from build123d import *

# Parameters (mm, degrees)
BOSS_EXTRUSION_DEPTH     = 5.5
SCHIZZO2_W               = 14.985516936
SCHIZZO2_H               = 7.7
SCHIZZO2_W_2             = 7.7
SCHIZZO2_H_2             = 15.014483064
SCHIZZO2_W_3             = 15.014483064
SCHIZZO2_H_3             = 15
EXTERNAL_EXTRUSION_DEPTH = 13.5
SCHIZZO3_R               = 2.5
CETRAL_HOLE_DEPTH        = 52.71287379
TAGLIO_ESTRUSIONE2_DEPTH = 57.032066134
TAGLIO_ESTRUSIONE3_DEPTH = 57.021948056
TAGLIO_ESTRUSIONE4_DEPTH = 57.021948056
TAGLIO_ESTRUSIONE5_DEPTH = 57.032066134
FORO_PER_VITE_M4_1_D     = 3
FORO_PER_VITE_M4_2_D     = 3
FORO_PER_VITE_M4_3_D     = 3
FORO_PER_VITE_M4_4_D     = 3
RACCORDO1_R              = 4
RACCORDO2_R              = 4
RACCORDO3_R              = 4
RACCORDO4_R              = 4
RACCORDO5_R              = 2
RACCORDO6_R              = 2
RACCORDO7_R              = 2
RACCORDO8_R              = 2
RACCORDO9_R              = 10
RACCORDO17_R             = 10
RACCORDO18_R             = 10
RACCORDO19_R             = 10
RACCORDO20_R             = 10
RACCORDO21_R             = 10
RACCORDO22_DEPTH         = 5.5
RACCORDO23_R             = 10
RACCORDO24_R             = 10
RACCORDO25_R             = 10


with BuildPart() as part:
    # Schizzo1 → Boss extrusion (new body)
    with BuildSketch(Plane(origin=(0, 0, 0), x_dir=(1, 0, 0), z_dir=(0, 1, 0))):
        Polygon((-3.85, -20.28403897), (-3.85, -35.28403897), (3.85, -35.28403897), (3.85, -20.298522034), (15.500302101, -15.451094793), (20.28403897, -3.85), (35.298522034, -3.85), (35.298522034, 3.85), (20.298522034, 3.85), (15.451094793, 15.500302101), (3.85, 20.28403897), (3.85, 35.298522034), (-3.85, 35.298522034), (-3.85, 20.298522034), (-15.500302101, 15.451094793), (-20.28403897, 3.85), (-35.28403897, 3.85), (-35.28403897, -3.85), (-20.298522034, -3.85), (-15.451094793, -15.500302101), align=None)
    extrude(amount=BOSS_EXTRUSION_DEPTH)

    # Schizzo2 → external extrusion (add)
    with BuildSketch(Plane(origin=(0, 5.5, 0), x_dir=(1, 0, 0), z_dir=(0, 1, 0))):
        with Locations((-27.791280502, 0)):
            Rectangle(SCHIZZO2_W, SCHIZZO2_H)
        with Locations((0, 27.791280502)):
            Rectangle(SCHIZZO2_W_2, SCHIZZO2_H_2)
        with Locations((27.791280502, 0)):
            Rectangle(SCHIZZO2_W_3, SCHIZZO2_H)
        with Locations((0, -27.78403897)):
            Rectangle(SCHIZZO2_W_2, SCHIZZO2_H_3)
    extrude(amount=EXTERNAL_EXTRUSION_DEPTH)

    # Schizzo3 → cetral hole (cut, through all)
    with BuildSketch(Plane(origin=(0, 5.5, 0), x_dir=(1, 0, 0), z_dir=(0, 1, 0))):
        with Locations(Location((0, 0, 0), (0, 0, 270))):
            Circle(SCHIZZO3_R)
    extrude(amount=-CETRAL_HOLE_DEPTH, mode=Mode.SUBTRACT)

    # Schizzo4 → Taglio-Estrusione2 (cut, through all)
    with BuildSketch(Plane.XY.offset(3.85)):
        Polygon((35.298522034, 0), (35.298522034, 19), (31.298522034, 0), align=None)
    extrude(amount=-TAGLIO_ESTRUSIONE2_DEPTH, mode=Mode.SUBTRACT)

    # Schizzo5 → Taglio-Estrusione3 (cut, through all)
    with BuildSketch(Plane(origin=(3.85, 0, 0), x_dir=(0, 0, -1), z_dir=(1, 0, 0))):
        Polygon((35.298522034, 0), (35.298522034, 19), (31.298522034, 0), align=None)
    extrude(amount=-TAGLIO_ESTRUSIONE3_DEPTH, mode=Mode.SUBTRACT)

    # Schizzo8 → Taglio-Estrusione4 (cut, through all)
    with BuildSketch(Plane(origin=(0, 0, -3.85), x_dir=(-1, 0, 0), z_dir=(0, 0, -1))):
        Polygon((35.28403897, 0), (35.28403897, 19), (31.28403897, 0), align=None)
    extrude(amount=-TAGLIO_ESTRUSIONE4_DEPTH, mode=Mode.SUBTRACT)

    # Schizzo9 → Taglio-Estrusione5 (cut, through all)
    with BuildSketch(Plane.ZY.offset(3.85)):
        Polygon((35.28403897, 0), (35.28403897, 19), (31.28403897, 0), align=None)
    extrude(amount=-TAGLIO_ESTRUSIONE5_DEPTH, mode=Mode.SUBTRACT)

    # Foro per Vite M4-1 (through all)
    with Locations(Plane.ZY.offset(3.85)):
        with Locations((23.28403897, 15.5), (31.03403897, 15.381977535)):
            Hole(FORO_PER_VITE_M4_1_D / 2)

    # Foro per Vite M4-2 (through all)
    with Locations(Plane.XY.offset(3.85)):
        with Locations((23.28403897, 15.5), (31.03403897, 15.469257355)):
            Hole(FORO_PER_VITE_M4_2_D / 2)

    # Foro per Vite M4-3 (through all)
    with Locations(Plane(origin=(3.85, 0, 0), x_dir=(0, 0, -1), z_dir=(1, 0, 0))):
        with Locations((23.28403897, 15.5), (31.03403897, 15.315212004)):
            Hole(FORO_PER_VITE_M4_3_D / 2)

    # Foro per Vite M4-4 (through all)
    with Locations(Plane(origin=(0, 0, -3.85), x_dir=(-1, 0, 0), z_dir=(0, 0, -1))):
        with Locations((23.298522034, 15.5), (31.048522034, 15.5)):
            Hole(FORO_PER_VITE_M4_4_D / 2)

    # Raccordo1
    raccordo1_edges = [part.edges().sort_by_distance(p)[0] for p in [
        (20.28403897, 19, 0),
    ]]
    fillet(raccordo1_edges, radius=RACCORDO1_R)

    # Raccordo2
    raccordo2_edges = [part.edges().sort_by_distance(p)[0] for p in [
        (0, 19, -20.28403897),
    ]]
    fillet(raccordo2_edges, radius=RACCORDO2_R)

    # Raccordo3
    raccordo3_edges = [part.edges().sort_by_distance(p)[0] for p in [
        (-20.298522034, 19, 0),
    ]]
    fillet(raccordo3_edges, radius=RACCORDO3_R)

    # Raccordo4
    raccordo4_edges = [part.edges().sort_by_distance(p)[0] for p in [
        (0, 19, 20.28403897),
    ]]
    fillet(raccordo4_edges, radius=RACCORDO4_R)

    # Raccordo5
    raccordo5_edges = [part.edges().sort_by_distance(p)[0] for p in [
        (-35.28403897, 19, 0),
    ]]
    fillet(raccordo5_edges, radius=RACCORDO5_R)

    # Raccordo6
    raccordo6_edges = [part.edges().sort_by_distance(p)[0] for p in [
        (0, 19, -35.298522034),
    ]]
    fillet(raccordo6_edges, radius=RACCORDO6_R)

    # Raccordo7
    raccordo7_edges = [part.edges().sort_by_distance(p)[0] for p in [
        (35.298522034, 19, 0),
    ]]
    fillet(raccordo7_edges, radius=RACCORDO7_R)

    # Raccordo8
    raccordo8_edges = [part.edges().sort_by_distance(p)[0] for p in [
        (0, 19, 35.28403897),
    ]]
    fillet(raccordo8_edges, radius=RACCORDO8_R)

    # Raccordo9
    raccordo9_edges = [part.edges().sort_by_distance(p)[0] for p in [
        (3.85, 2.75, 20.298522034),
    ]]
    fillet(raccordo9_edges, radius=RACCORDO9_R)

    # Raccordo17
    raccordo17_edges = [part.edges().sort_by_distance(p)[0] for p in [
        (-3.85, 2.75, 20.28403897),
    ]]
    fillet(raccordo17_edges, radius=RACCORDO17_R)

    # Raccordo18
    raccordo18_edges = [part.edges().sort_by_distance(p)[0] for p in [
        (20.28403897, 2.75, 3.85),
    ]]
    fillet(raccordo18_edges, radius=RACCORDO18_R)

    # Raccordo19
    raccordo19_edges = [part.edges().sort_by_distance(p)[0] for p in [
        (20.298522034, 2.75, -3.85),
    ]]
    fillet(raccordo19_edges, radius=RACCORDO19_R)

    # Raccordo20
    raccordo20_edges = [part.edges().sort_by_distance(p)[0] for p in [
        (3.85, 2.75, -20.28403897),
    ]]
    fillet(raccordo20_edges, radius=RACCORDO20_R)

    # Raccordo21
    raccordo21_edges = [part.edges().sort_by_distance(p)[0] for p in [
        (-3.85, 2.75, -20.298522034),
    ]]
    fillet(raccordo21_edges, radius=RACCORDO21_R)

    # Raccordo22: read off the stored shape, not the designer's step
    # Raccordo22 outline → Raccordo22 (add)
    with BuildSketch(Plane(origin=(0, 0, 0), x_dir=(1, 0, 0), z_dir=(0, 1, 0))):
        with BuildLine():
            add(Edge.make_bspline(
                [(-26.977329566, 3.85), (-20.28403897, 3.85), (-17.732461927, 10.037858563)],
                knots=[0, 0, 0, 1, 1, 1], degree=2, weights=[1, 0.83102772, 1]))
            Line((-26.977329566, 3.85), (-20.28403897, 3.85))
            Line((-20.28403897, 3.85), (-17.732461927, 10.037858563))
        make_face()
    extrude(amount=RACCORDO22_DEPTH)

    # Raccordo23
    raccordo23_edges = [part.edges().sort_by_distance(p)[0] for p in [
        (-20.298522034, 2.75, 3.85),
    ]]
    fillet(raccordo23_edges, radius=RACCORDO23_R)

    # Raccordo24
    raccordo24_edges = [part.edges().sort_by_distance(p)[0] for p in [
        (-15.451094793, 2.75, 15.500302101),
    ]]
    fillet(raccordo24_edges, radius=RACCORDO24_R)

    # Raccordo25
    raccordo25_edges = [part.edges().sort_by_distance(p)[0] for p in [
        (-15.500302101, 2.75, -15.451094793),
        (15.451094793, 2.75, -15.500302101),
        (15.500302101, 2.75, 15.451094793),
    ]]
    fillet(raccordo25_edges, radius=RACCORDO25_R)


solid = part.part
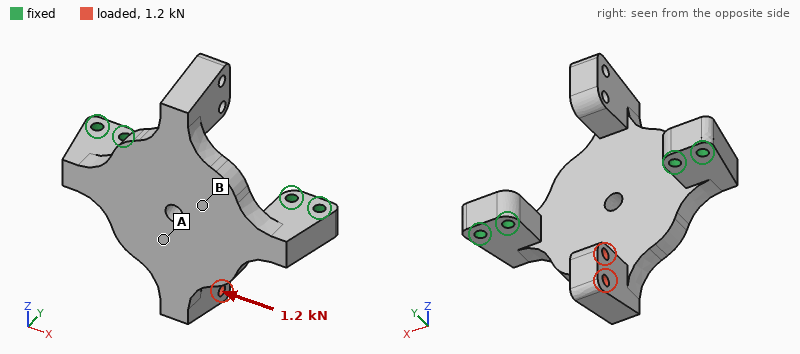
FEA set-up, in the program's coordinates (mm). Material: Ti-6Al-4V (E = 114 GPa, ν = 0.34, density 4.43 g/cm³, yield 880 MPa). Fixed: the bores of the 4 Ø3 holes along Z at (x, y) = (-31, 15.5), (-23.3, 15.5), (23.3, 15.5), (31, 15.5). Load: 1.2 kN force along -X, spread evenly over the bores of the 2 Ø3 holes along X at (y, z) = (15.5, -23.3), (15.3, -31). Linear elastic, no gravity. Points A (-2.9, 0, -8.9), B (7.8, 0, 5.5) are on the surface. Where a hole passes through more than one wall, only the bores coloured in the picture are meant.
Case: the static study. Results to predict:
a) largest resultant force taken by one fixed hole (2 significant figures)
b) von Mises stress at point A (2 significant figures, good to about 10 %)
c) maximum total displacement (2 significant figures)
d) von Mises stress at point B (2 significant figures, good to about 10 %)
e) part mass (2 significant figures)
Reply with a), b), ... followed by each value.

a) 1.2 kN
b) 78 MPa
c) 0.18 mm
d) 30 MPa
e) 64 g
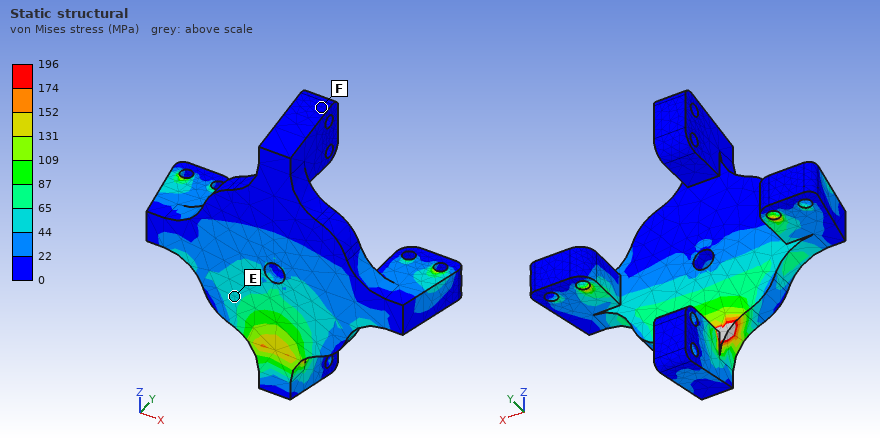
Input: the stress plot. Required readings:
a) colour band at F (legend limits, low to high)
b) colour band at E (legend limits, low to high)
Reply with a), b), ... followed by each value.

a) 0 to 22 MPa
b) 44 to 65 MPa
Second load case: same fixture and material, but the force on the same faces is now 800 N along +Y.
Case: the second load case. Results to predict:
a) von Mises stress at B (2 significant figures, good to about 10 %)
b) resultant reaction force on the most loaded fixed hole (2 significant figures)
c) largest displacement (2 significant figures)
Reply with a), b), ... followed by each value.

a) 31 MPa
b) 420 N
c) 0.42 mm
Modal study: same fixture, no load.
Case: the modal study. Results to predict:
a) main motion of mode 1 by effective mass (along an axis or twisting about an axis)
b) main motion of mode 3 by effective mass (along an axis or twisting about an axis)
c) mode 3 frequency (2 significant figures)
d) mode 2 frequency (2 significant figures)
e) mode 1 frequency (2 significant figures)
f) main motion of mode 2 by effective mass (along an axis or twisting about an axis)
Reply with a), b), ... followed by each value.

a) twisting about X
b) twisting about Y
c) 6500 Hz
d) 3500 Hz
e) 2200 Hz
f) along Y
